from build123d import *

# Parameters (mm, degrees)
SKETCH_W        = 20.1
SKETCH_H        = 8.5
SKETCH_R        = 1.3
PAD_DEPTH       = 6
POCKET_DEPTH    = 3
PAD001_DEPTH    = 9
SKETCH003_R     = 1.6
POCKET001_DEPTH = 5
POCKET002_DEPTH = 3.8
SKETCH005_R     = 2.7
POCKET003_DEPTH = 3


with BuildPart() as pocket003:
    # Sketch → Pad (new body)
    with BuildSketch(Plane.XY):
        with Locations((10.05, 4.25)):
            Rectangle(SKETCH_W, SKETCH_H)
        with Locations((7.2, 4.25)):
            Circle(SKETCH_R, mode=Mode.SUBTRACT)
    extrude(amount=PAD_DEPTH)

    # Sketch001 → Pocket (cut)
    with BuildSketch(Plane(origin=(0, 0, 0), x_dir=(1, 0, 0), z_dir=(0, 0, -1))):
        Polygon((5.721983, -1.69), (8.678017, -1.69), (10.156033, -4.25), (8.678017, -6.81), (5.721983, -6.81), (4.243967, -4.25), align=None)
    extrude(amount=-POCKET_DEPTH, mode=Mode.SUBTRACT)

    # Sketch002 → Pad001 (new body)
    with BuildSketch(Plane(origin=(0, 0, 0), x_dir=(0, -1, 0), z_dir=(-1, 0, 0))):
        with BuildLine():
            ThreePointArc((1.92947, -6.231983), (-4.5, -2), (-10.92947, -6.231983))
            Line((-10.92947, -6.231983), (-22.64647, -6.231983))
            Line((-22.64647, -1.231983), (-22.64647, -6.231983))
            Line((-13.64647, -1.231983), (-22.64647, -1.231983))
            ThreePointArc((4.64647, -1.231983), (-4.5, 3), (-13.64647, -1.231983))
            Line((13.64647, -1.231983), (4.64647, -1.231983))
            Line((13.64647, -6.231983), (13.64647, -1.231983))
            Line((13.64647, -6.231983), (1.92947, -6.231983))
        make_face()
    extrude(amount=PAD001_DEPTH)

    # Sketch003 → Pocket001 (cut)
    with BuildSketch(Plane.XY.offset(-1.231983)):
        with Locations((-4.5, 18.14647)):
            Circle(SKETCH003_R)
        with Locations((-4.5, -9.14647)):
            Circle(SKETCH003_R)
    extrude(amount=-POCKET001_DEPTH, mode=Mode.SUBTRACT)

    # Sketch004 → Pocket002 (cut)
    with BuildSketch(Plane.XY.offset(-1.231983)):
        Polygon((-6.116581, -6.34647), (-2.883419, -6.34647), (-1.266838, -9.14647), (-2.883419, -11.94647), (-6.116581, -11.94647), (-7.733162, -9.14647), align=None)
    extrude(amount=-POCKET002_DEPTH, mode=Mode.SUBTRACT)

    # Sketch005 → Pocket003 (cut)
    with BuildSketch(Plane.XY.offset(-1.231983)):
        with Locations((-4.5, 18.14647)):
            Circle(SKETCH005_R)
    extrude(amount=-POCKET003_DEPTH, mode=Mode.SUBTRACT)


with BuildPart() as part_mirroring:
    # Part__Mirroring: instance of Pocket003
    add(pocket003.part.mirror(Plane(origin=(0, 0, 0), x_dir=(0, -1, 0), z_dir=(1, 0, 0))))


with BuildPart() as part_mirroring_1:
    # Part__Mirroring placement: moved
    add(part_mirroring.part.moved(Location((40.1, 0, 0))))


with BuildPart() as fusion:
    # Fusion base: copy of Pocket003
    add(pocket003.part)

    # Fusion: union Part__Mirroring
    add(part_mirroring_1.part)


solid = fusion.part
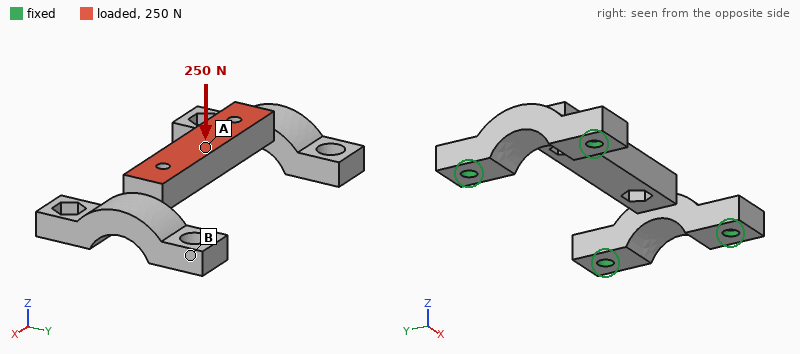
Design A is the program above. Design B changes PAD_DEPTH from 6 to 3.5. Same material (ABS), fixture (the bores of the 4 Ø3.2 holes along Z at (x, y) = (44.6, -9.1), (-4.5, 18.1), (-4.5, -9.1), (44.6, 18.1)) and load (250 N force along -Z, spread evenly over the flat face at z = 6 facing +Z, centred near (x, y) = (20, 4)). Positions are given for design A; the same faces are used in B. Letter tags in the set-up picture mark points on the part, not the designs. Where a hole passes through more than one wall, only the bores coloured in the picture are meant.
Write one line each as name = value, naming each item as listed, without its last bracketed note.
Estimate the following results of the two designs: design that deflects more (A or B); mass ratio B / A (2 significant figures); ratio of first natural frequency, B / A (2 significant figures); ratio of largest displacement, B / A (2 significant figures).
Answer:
design that deflects more = B
mass ratio B / A = 0.84
ratio of first natural frequency, B / A = 0.83
ratio of largest displacement, B / A = 2.6
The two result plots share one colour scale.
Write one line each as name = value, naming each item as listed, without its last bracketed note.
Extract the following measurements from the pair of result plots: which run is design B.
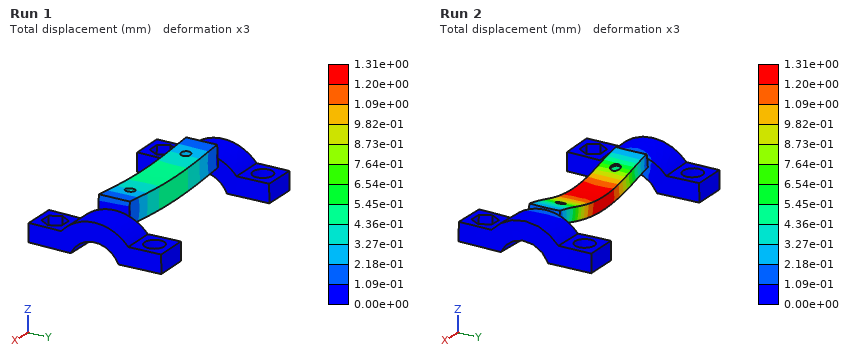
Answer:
which run is design B = Run 2
